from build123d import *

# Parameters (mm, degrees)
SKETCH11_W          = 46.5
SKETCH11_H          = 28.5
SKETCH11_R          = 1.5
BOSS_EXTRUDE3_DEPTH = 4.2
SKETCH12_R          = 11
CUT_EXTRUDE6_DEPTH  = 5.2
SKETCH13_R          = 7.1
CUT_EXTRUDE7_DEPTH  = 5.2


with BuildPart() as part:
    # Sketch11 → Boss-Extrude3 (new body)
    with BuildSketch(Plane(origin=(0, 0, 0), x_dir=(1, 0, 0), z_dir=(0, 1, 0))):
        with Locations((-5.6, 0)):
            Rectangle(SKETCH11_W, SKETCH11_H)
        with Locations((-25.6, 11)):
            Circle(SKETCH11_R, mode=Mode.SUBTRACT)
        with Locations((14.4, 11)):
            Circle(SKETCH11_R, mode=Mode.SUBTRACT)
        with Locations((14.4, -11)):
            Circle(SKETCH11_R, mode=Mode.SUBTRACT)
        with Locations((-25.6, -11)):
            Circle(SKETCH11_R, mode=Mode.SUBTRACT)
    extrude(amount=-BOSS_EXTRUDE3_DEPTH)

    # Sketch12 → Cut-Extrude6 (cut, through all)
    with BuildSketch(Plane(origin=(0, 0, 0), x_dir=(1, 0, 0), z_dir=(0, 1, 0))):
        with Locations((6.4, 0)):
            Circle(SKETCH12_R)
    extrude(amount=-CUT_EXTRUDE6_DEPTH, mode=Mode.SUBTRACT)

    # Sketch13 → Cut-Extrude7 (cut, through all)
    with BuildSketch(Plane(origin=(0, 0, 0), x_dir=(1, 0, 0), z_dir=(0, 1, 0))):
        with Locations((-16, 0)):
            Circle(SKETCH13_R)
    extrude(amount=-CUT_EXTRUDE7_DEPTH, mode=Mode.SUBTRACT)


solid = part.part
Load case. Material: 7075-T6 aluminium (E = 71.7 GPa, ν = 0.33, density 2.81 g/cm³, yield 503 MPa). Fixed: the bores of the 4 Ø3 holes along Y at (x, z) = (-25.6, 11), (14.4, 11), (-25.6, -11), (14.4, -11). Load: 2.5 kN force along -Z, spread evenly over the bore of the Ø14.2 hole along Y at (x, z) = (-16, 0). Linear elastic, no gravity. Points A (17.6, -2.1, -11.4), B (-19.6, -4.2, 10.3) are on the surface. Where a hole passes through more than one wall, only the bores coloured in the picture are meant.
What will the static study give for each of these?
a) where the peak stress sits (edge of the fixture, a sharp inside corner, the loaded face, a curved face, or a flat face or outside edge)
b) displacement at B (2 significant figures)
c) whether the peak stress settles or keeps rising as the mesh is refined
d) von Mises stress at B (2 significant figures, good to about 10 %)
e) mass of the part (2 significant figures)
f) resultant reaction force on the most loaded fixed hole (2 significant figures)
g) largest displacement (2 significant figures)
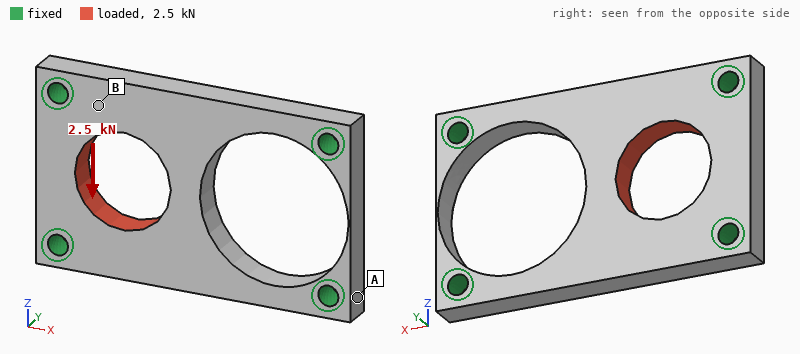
edge of the fixture
8.7 µm
keeps rising
44 MPa
9.0 g
1.2 kN
27 µm
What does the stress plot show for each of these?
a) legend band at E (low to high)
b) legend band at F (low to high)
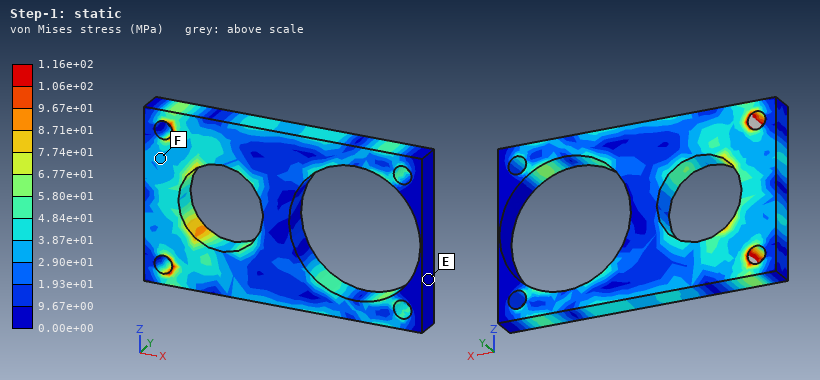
0.00e+00 to 9.67e+00 MPa
2.90e+01 to 3.87e+01 MPa
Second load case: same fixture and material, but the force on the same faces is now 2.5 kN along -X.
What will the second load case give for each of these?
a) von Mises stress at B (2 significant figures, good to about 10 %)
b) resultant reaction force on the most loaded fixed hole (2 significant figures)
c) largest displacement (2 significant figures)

33 MPa
1.1 kN
11 µm
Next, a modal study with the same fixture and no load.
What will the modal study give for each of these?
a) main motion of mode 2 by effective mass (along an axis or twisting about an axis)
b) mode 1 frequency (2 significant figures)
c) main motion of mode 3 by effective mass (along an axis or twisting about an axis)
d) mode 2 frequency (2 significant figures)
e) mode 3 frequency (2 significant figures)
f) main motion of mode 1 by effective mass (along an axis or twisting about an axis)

twisting about X
11 kHz
along Z
15 kHz
18 kHz
along Y
